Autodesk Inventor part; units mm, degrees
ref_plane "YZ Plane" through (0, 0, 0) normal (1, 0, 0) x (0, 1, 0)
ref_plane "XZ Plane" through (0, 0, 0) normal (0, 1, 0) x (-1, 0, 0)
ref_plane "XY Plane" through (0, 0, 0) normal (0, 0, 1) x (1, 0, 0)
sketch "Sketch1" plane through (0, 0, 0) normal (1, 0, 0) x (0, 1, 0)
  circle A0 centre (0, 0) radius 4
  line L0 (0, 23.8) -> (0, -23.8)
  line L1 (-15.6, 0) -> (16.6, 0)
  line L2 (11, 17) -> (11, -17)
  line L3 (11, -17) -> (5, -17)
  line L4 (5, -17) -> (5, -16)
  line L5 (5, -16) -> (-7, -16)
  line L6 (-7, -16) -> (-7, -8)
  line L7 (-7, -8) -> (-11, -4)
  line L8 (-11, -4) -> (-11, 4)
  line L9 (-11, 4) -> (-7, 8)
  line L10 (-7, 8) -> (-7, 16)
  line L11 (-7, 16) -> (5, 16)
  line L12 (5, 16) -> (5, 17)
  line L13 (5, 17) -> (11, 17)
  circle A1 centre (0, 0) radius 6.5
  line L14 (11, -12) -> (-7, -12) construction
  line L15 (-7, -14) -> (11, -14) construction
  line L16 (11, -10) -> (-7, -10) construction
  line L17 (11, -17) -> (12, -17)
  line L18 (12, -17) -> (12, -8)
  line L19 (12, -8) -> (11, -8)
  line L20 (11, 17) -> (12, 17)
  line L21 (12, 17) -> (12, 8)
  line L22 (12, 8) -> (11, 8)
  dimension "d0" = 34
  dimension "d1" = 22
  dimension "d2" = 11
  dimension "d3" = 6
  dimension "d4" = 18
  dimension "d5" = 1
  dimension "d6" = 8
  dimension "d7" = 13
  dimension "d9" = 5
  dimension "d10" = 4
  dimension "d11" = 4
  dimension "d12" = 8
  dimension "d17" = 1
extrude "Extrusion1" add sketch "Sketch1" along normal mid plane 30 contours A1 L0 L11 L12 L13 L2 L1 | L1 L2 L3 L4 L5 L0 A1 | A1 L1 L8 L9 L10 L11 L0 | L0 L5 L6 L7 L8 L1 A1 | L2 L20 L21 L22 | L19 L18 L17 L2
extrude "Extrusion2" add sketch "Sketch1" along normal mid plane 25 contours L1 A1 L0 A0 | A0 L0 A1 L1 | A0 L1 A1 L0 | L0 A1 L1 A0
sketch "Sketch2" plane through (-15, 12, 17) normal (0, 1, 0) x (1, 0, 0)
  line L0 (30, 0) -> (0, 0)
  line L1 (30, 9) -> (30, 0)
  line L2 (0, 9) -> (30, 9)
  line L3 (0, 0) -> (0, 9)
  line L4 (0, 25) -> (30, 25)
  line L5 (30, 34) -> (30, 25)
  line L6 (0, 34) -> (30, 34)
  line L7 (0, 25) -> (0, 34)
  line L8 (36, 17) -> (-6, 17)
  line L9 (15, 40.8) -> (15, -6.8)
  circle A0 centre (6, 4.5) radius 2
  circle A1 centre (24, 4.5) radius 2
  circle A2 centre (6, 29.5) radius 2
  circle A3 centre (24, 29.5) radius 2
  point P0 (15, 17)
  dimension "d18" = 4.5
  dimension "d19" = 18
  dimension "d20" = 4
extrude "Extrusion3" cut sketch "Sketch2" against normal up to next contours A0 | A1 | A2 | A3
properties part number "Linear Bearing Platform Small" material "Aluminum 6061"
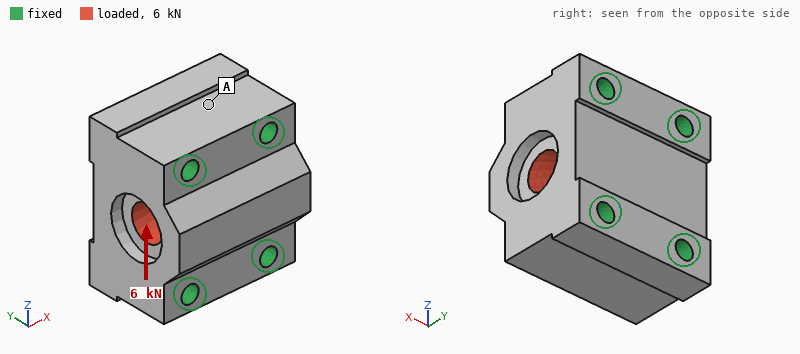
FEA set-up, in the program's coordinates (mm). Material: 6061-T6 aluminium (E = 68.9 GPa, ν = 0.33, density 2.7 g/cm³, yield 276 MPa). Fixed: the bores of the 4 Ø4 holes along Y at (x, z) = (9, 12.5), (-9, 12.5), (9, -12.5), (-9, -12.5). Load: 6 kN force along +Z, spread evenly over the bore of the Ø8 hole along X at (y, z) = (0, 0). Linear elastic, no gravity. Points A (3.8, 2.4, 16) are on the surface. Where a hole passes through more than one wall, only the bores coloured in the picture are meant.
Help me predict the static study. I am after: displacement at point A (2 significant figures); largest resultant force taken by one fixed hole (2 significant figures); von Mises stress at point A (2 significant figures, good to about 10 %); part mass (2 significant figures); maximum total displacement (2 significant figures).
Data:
0.57 µm
1.5 kN
2.5 MPa
45 g
1.9 µm
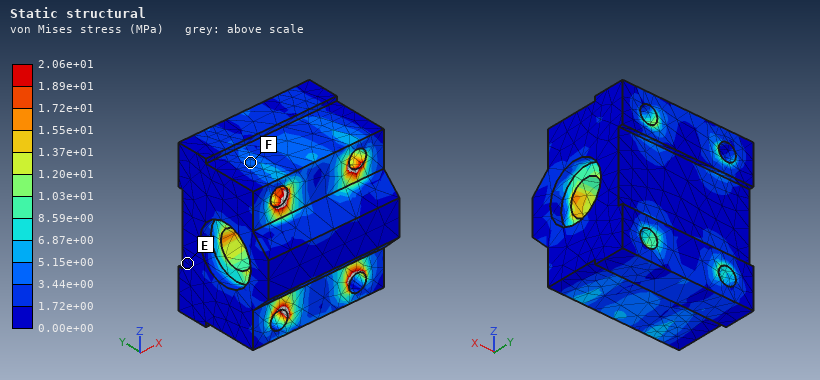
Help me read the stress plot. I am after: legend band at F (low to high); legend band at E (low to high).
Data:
3.44e+00 to 5.15e+00 MPa
0.00e+00 to 1.72e+00 MPa
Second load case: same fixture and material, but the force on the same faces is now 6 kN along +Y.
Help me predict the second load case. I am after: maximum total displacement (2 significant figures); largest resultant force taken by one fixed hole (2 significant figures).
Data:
3.5 µm
1.5 kN
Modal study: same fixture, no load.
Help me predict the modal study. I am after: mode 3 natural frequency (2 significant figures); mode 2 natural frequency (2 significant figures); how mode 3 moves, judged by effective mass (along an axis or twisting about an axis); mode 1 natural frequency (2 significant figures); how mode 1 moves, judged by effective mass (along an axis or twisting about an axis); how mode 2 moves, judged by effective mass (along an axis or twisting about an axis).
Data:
63 kHz
55 kHz
along X
51 kHz
along X
along Y
